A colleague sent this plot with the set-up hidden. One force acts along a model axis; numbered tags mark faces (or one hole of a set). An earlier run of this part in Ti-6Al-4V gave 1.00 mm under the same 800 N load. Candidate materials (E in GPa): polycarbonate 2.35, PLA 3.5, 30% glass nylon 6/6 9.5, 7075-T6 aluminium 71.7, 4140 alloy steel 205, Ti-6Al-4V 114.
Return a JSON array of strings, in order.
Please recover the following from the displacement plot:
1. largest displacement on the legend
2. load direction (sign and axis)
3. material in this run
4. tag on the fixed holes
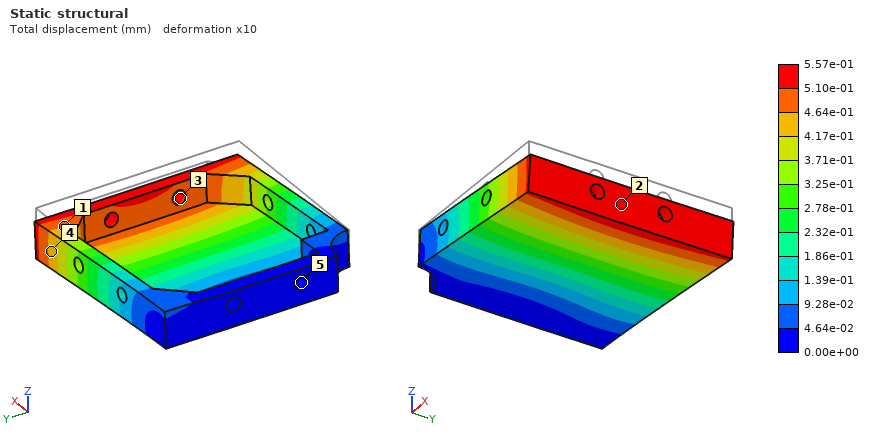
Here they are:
["5.57e-01 mm", "-Z", "4140 alloy steel", "5"]
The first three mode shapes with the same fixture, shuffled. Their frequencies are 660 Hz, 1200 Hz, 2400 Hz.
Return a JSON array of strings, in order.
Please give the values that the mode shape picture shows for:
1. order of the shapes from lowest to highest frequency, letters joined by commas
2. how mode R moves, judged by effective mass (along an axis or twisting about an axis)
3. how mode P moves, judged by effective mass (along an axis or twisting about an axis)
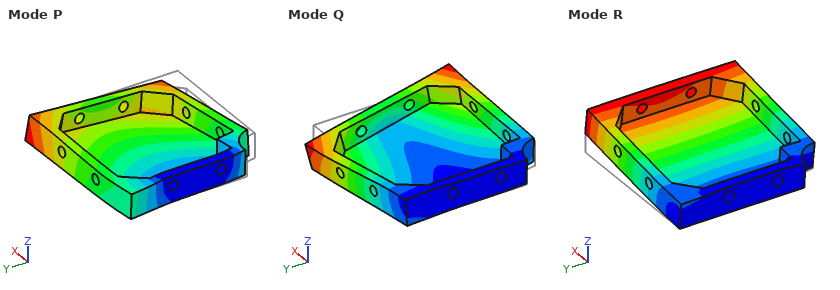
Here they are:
["R, Q, P", "along Z", "along Y"]
